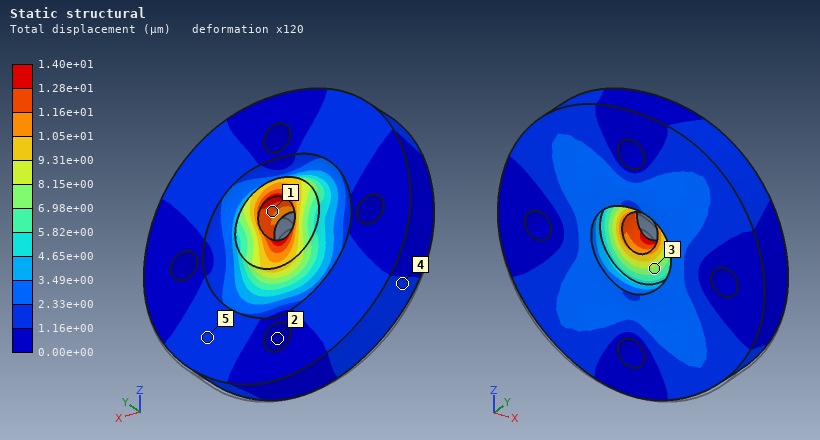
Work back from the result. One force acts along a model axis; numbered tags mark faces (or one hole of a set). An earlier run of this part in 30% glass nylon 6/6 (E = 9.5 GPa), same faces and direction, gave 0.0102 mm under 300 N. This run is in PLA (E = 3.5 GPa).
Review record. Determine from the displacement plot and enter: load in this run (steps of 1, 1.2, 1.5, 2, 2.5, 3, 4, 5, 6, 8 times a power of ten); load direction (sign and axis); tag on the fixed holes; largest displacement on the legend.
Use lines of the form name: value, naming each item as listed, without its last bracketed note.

load in this run: 150 N
load direction: +Z
tag on the fixed holes: 2
largest displacement on the legend: 1.40e+01 µm
